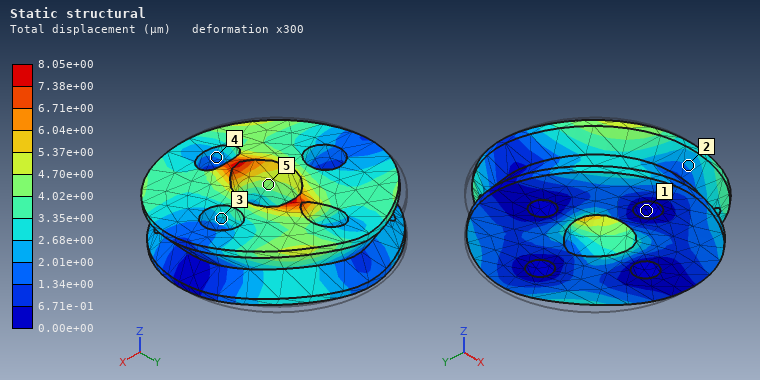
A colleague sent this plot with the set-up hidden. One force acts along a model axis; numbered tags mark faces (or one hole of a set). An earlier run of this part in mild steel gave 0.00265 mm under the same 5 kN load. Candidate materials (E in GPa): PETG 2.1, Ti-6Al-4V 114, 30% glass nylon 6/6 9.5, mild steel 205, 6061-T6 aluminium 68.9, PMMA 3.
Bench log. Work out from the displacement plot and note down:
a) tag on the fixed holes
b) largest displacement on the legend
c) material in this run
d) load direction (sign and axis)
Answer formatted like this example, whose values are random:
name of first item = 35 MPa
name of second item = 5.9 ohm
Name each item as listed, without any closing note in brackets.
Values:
tag on the fixed holes = 1
largest displacement on the legend = 8.05e+00 µm
material in this run = 6061-T6 aluminium
load direction = -Y
